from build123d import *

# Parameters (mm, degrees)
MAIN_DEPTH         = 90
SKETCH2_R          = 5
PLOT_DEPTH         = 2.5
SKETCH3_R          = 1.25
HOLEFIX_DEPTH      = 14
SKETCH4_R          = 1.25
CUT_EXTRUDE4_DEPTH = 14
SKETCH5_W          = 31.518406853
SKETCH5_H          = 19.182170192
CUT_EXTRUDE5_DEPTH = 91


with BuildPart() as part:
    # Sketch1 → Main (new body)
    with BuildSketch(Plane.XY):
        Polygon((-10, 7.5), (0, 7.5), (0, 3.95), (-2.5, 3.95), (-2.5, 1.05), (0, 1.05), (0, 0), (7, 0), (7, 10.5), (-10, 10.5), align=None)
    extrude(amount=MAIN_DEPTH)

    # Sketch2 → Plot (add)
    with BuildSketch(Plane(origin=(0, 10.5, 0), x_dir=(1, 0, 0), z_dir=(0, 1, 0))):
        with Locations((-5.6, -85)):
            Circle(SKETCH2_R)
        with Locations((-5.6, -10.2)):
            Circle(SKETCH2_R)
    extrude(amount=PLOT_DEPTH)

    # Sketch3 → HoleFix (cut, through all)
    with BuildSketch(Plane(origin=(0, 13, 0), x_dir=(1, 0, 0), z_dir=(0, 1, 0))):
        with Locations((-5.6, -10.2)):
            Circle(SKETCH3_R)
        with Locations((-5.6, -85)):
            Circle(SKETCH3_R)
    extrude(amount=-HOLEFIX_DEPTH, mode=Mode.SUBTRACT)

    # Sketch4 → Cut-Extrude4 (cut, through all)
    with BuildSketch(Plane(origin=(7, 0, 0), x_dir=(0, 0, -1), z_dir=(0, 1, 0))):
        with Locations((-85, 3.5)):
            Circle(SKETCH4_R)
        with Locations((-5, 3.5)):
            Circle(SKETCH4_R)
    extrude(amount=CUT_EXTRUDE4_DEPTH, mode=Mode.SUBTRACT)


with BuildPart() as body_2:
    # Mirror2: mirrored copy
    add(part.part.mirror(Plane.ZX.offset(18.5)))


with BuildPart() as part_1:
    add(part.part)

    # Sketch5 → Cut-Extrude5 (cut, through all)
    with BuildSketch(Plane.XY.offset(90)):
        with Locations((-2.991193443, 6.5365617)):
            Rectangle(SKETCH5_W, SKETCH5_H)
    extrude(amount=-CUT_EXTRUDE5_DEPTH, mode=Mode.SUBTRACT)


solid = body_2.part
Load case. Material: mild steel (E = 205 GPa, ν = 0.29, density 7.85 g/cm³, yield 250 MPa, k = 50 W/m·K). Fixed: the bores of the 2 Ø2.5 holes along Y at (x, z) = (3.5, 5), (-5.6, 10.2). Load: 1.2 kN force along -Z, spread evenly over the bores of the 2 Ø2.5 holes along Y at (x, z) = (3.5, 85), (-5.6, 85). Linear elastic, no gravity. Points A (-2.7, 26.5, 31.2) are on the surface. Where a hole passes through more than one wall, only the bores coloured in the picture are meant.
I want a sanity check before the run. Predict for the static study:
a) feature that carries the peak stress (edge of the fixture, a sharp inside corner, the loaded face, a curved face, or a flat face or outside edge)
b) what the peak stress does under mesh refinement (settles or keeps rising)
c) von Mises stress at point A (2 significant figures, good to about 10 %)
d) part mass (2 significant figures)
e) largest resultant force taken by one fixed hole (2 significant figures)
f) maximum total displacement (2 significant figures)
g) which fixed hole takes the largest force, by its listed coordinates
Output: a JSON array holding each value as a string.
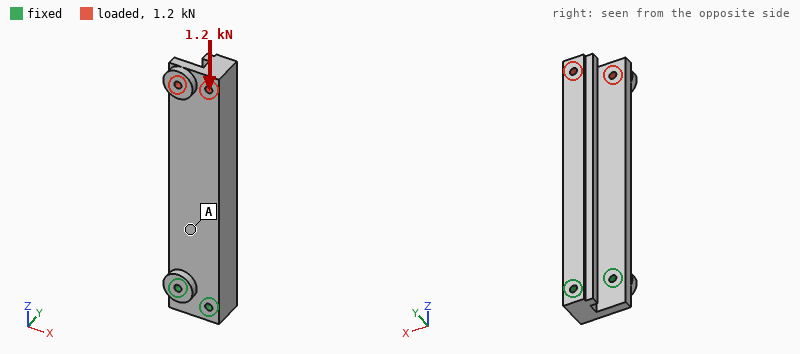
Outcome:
["edge of the fixture", "keeps rising", "15 MPa", "80 g", "780 N", "17 µm", "(3.5, 5)"]
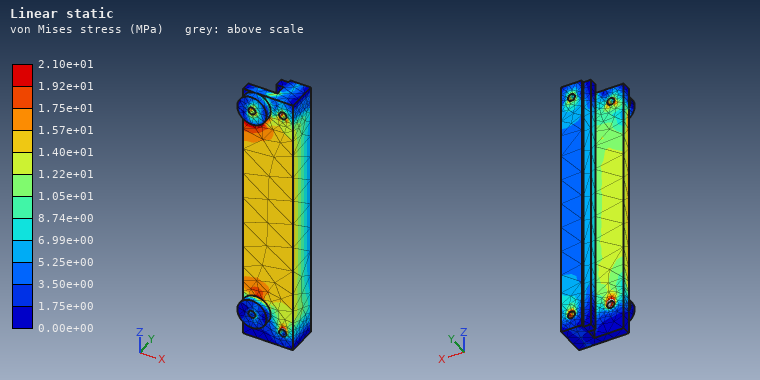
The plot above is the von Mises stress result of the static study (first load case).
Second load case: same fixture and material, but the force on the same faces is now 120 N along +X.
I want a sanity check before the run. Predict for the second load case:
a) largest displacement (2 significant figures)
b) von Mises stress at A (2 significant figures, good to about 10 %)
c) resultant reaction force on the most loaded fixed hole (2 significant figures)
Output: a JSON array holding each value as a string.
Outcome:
["70 µm", "5.8 MPa", "740 N"]
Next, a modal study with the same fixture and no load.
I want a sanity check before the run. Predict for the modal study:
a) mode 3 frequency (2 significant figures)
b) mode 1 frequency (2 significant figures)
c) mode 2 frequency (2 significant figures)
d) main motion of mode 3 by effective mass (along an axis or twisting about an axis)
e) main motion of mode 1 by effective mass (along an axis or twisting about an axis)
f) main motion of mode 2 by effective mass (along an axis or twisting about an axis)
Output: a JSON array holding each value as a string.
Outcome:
["5000 Hz", "1000 Hz", "1900 Hz", "twisting about Z", "along Y", "along X"]
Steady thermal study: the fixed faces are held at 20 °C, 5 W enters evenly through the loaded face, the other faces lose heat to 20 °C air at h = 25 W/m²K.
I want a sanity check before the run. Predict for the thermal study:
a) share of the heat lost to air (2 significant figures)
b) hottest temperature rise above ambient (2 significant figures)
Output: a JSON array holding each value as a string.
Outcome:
["53 %", "43 K"]
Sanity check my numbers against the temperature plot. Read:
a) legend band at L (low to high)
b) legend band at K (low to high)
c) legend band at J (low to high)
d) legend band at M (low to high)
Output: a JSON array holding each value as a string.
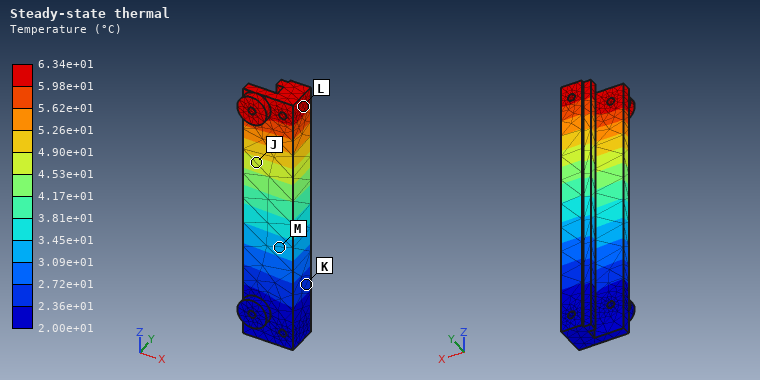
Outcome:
["5.98e+01 to 6.34e+01 °C", "2.36e+01 to 2.72e+01 °C", "4.53e+01 to 4.90e+01 °C", "3.09e+01 to 3.45e+01 °C"]
